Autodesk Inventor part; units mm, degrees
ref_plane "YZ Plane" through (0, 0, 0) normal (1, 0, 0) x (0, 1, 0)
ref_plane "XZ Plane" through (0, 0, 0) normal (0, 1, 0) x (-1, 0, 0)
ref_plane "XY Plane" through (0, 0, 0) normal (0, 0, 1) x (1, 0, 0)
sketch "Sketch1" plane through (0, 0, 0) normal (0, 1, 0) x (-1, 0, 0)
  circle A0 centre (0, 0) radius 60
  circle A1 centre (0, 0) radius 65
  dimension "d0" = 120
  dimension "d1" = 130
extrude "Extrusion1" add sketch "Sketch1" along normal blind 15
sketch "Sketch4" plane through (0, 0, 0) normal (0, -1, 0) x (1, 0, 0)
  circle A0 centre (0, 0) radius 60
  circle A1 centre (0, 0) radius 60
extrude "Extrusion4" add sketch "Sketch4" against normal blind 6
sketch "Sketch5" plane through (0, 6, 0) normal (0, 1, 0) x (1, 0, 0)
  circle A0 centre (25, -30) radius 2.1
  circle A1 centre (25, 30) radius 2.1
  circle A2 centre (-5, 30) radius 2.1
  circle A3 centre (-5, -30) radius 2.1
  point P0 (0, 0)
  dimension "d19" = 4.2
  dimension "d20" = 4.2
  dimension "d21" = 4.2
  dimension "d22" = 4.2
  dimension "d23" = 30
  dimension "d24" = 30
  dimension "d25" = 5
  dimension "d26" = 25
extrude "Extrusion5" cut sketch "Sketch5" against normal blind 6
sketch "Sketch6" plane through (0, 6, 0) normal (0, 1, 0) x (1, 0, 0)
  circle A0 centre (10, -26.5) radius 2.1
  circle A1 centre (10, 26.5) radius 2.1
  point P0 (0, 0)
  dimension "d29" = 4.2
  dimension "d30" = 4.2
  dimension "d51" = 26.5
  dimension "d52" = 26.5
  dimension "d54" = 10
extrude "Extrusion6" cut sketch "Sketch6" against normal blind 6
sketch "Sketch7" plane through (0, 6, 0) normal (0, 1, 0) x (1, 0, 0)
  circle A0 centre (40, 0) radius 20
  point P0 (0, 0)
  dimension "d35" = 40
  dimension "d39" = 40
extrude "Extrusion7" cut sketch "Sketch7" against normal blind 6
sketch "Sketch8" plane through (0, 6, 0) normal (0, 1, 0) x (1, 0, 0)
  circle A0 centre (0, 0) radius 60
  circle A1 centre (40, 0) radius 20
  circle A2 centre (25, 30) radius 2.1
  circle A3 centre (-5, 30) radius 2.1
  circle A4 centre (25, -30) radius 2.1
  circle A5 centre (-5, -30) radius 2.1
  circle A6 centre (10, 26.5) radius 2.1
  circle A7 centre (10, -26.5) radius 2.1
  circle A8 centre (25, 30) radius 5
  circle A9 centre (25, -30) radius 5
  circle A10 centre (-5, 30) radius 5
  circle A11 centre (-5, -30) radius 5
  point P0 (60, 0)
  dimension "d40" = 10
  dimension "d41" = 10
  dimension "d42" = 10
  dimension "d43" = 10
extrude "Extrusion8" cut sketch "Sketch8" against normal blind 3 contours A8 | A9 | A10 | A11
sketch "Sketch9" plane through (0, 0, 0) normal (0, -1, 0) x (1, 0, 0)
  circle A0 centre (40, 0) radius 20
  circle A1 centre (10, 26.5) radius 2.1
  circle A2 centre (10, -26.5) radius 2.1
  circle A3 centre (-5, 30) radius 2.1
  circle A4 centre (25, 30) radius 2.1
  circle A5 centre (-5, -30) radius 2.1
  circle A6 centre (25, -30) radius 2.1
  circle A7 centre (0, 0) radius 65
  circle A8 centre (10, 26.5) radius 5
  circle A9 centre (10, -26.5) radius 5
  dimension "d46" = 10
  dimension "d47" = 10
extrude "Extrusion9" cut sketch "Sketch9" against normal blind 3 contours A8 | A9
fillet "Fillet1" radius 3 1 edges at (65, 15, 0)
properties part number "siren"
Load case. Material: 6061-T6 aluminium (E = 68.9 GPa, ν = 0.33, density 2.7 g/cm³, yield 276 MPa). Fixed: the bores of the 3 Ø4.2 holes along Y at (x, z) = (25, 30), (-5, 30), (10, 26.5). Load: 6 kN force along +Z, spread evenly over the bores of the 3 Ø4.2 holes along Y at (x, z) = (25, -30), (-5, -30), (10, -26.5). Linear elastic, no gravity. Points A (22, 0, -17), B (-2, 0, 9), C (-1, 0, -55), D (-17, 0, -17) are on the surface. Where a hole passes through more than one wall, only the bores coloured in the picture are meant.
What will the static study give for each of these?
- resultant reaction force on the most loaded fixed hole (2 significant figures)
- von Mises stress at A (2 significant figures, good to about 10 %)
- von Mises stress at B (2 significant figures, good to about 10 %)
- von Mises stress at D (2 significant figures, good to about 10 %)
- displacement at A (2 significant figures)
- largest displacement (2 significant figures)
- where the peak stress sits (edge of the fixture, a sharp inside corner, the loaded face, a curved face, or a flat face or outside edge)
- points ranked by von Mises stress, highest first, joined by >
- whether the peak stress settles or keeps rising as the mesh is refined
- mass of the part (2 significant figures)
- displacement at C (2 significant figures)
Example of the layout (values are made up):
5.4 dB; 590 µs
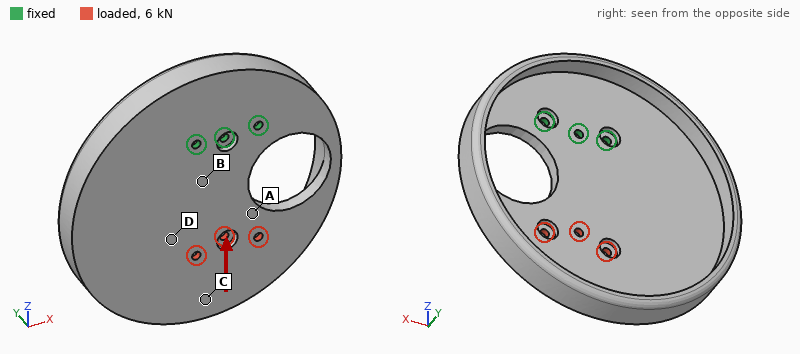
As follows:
2.1 kN; 31 MPa; 21 MPa; 13 MPa; 38 µm; 93 µm; edge of the fixture; A > B > D > C; keeps rising; 240 g; 79 µm
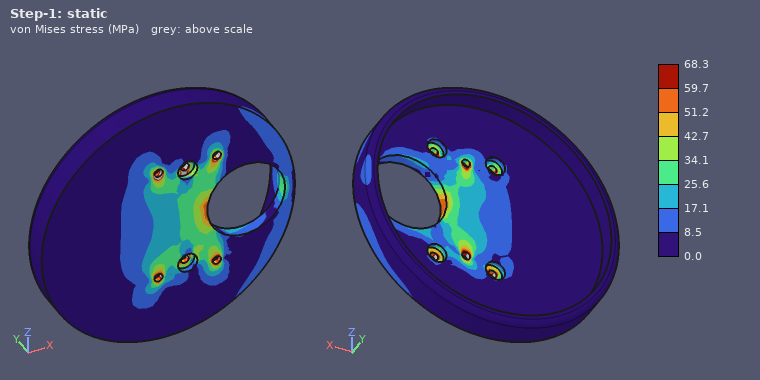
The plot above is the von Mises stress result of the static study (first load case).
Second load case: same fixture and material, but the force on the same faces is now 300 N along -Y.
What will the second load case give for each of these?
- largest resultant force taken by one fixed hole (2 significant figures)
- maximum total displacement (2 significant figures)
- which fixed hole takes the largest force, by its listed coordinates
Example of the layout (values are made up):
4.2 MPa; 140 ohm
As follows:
1.9 kN; 0.39 mm; (10, 26.5)
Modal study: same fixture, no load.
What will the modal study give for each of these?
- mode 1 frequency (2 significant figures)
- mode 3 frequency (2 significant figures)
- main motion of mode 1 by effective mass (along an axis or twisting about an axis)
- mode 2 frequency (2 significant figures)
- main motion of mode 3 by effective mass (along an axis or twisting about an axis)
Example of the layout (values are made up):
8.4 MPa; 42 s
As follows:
460 Hz; 2000 Hz; along Y; 1000 Hz; along X
